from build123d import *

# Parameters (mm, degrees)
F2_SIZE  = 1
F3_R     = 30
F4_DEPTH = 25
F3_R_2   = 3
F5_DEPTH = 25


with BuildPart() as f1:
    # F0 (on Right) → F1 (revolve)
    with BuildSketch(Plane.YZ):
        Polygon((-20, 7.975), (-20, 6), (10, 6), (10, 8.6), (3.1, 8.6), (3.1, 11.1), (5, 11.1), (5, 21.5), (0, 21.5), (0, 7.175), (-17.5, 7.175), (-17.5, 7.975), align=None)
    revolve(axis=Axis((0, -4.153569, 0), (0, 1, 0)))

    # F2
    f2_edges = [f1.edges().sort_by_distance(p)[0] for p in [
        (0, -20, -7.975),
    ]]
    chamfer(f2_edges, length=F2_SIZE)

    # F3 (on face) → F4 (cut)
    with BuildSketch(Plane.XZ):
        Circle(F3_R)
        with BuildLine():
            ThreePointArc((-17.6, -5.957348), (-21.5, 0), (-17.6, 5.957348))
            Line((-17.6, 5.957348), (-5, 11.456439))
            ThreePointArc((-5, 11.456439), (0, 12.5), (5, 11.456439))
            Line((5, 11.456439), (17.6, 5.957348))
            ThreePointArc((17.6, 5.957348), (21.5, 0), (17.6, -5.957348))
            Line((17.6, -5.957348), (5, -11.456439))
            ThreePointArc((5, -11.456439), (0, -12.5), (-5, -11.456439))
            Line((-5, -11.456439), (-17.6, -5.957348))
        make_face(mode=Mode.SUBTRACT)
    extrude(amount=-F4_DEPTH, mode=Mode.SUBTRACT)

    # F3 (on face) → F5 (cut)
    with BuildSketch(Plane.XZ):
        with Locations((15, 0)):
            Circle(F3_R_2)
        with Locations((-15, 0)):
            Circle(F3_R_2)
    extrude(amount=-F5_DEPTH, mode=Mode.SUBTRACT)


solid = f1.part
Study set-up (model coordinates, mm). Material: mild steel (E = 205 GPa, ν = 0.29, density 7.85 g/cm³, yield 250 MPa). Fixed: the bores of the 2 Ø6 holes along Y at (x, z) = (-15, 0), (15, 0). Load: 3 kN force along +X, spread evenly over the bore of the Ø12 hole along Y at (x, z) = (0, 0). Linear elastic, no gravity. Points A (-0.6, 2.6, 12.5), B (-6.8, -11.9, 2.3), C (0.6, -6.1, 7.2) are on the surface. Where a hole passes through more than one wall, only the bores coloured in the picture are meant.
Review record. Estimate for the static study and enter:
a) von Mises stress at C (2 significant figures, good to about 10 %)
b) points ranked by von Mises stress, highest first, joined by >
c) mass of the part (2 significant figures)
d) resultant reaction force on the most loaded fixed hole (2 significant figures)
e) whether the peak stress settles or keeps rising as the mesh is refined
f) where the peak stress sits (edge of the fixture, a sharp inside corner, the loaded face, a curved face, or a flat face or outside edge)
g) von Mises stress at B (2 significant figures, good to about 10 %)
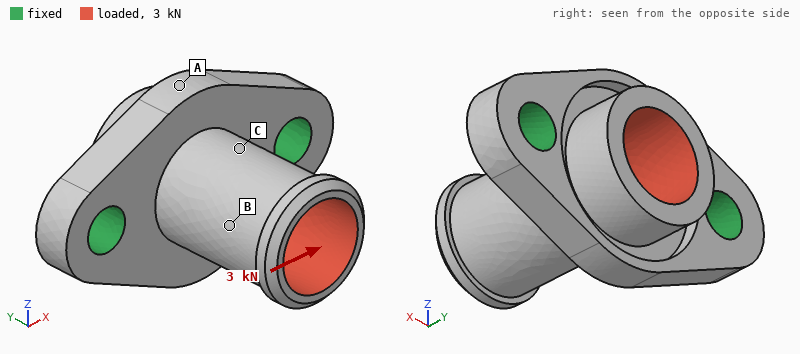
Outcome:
95 MPa
C > B > A
33 g
1.8 kN
keeps rising
a sharp inside corner
31 MPa
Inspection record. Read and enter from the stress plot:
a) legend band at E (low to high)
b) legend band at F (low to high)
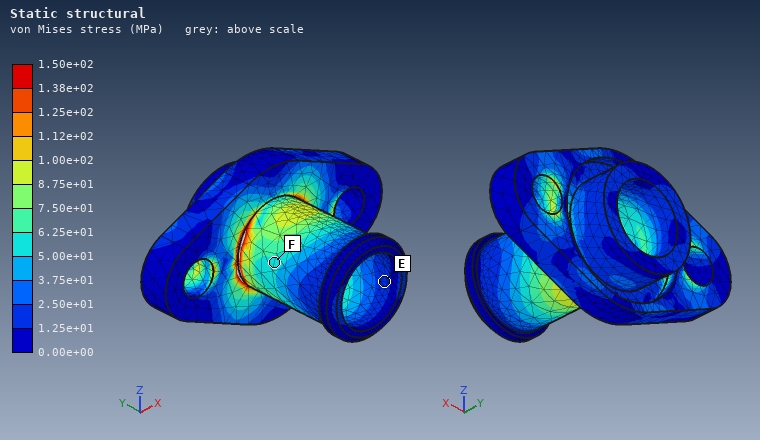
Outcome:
1.25e+01 to 2.50e+01 MPa
5.00e+01 to 6.25e+01 MPa
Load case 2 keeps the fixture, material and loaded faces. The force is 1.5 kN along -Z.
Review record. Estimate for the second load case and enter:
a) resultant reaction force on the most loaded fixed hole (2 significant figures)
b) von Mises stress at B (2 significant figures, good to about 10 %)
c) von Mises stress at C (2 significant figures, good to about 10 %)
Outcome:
750 N
25 MPa
33 MPa
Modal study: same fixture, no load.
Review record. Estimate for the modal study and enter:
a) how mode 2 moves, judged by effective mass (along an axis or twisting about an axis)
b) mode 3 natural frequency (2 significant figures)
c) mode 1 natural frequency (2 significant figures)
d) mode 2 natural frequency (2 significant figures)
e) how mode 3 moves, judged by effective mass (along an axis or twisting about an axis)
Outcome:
along X
19 kHz
9100 Hz
14 kHz
along Y
